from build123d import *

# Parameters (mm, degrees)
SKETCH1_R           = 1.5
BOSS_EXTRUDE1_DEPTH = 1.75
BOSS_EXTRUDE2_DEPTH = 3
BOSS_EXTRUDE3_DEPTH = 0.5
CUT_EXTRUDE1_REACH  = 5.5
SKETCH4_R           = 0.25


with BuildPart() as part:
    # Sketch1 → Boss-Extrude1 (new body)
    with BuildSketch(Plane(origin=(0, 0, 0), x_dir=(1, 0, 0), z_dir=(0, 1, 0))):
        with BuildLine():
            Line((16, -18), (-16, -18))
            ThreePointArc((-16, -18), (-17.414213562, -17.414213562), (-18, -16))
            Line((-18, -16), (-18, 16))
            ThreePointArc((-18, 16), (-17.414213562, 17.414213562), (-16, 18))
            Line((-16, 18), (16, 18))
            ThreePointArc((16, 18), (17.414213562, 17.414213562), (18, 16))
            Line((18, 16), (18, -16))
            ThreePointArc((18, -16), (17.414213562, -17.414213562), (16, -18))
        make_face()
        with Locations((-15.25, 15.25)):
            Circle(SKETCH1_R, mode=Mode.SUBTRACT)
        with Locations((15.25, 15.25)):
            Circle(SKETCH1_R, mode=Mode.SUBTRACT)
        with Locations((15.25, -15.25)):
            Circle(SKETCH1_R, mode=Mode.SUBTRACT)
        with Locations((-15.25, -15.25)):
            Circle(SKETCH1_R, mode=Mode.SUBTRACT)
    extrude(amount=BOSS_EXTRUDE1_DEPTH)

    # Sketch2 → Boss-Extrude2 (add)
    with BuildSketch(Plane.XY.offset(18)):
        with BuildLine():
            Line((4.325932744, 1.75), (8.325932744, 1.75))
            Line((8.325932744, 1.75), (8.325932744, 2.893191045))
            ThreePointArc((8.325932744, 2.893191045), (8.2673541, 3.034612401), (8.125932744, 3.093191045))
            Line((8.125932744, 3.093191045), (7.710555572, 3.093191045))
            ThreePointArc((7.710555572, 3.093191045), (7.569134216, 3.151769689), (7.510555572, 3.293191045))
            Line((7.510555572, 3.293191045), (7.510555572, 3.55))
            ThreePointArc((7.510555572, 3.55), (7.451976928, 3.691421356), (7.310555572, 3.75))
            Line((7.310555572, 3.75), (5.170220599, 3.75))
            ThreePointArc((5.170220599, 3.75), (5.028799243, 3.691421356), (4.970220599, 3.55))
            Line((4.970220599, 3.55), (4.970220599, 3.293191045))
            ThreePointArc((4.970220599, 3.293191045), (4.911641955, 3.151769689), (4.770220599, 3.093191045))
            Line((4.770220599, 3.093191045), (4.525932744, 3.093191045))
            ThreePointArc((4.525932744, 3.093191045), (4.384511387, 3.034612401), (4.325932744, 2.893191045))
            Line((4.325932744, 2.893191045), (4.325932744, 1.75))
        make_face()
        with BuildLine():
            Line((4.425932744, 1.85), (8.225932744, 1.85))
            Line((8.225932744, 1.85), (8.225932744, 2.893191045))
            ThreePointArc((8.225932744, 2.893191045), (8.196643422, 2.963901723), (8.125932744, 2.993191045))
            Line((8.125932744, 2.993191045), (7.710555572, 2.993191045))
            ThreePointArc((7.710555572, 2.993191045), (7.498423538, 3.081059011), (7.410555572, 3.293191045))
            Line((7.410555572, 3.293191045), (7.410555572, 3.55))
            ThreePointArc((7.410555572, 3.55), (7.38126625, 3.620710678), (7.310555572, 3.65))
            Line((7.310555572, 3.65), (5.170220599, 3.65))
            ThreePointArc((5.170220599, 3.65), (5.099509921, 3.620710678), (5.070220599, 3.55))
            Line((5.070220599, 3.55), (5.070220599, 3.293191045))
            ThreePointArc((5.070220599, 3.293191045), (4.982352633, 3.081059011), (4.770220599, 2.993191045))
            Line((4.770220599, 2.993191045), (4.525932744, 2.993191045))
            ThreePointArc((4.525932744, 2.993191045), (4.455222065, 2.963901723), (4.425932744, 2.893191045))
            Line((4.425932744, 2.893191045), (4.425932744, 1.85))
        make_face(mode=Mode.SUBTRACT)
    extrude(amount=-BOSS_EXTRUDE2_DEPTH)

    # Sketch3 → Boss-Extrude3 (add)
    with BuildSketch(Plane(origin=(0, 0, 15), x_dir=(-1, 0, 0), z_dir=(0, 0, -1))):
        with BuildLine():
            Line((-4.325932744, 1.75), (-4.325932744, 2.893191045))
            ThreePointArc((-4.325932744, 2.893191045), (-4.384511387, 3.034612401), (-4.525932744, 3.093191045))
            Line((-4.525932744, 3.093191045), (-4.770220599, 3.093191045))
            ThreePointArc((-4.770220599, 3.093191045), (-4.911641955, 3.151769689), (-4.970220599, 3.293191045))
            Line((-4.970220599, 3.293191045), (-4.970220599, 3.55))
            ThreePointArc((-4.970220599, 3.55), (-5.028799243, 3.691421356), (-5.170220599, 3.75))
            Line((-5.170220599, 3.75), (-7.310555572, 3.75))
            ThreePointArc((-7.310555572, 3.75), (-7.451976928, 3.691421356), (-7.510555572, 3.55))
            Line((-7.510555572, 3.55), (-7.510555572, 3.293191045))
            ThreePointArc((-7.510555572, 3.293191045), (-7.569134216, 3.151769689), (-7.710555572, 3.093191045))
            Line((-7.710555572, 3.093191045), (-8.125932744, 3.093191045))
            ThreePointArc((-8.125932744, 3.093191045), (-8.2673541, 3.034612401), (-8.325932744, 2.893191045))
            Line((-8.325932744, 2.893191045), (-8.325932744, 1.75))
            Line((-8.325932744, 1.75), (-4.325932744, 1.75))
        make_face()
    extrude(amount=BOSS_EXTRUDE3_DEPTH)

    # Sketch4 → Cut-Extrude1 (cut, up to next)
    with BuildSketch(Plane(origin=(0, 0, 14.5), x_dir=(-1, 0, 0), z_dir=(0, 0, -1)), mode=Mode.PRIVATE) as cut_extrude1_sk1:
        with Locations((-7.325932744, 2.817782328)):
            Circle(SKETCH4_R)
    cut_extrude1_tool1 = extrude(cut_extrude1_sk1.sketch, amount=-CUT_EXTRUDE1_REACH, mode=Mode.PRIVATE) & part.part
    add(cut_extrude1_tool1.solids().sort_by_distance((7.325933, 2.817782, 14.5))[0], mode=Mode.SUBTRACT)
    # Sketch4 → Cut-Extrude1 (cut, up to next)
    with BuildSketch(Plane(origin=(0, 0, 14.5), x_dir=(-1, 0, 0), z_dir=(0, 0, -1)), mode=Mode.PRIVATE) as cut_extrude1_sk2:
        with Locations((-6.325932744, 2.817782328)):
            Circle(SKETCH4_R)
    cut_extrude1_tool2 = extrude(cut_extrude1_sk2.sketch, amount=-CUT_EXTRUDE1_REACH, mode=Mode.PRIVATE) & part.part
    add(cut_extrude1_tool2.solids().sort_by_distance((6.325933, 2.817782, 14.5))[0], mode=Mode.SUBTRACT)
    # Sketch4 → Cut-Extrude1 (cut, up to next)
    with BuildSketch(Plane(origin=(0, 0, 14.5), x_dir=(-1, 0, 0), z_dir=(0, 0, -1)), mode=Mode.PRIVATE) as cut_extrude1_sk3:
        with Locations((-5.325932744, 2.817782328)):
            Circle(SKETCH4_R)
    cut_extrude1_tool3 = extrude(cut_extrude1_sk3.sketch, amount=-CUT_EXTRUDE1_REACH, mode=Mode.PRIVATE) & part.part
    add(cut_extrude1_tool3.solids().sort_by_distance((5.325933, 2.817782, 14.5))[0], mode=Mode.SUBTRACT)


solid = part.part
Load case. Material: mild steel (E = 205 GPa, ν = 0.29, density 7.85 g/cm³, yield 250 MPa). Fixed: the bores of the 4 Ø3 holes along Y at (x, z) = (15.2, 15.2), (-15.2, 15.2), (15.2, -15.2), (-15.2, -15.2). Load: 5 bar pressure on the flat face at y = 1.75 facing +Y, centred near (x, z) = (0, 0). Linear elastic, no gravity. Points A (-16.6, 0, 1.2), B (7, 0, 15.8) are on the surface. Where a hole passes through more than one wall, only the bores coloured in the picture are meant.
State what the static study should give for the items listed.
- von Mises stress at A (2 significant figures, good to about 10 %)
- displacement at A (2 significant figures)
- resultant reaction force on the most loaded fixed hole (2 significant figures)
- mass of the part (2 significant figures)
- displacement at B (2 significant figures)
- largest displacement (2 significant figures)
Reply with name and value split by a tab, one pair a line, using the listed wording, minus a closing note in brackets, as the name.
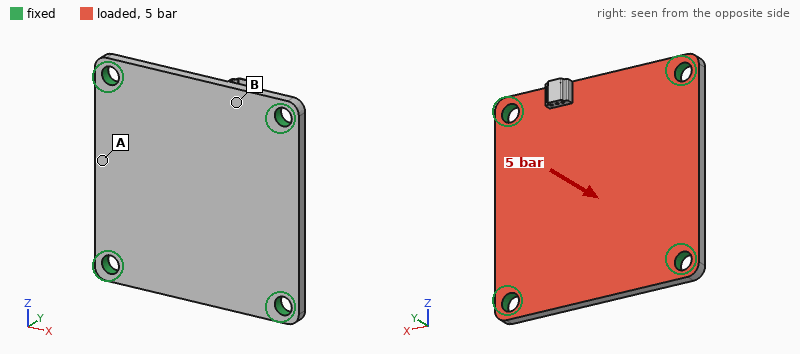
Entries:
von Mises stress at A	46 MPa
displacement at A	13 µm
resultant reaction force on the most loaded fixed hole	160 N
mass of the part	17 g
displacement at B	7.7 µm
largest displacement	28 µm
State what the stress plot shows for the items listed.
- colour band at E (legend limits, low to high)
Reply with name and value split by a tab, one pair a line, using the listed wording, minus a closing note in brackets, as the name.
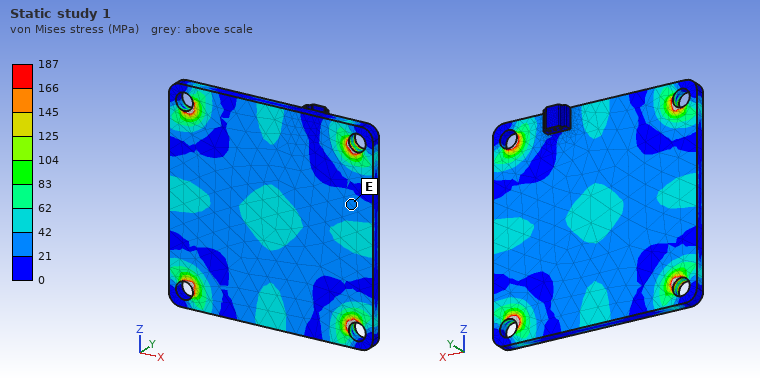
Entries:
colour band at E	21 to 42 MPa
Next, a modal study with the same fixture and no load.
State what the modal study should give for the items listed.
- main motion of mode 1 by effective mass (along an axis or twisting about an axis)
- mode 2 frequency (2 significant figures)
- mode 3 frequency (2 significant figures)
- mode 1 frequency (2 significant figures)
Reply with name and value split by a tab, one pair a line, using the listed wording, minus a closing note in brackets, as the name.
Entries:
main motion of mode 1 by effective mass	along Y
mode 2 frequency	12 kHz
mode 3 frequency	12 kHz
mode 1 frequency	7000 Hz
